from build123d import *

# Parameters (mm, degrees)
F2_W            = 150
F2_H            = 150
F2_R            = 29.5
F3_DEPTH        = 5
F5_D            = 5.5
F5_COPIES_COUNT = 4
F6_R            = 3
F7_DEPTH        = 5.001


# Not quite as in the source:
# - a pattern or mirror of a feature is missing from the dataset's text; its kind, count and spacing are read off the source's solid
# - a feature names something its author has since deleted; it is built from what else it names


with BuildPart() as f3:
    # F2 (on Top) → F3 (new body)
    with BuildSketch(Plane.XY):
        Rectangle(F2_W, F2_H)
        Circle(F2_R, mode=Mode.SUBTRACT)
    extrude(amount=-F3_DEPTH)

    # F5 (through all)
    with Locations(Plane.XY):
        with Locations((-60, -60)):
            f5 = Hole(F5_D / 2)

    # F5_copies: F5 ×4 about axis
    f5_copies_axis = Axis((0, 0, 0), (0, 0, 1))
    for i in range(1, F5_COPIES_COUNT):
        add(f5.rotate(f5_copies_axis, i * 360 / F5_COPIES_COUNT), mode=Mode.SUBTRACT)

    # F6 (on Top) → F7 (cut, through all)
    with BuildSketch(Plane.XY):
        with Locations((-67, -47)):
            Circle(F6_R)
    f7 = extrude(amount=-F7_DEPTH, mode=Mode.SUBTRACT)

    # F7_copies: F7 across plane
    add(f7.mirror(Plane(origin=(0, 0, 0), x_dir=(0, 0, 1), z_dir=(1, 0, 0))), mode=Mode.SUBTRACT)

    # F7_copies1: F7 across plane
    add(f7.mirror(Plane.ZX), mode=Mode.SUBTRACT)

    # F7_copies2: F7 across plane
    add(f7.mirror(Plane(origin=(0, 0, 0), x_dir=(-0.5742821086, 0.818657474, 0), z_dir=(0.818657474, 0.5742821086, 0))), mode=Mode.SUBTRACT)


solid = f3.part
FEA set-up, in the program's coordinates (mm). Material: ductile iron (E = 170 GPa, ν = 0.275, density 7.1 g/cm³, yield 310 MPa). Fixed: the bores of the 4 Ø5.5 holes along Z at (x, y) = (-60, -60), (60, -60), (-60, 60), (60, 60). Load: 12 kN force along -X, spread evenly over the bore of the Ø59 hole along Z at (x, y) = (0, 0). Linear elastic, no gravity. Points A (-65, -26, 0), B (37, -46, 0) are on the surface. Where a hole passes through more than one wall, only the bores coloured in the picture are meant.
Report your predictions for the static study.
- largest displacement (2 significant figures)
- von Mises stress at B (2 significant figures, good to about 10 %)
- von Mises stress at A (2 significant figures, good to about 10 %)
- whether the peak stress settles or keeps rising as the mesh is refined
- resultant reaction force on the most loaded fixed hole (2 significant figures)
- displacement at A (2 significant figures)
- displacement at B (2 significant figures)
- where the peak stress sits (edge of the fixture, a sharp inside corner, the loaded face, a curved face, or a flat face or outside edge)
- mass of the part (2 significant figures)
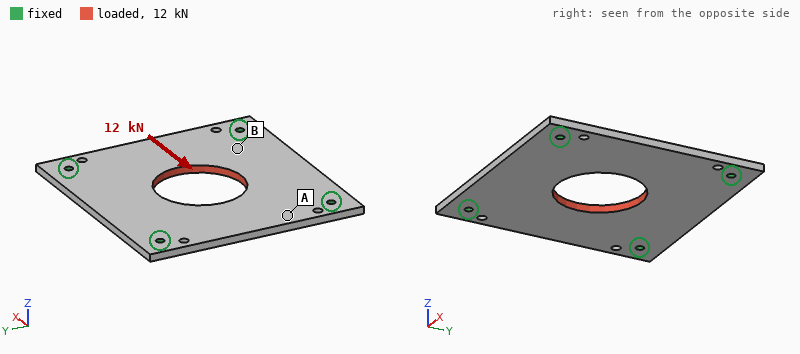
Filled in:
10 µm
17 MPa
7.5 MPa
keeps rising
3.2 kN
7.1 µm
4.3 µm
edge of the fixture
690 g
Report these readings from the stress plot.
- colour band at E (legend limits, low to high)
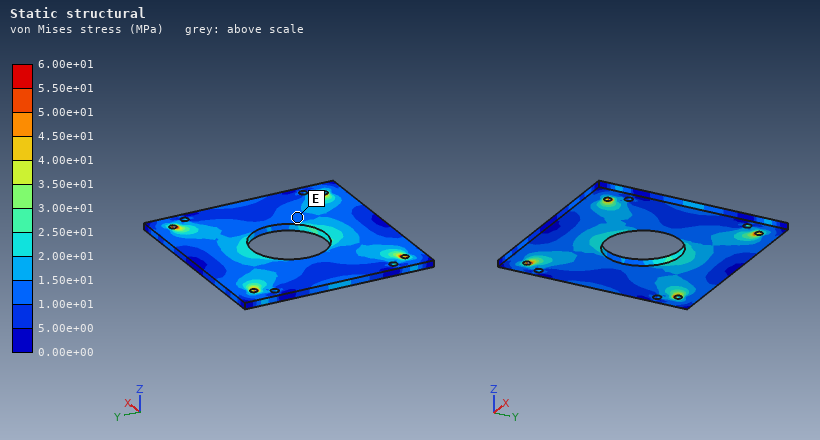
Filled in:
1.00e+01 to 1.50e+01 MPa
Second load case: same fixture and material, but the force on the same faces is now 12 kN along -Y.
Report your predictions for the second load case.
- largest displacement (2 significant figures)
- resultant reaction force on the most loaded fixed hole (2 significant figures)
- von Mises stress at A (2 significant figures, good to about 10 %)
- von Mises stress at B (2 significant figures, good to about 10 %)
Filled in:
11 µm
3.2 kN
9.1 MPa
16 MPa
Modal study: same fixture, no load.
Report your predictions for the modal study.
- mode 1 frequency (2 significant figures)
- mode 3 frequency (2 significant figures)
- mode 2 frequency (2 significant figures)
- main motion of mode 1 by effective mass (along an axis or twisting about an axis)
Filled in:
1200 Hz
1800 Hz
1800 Hz
along Z
